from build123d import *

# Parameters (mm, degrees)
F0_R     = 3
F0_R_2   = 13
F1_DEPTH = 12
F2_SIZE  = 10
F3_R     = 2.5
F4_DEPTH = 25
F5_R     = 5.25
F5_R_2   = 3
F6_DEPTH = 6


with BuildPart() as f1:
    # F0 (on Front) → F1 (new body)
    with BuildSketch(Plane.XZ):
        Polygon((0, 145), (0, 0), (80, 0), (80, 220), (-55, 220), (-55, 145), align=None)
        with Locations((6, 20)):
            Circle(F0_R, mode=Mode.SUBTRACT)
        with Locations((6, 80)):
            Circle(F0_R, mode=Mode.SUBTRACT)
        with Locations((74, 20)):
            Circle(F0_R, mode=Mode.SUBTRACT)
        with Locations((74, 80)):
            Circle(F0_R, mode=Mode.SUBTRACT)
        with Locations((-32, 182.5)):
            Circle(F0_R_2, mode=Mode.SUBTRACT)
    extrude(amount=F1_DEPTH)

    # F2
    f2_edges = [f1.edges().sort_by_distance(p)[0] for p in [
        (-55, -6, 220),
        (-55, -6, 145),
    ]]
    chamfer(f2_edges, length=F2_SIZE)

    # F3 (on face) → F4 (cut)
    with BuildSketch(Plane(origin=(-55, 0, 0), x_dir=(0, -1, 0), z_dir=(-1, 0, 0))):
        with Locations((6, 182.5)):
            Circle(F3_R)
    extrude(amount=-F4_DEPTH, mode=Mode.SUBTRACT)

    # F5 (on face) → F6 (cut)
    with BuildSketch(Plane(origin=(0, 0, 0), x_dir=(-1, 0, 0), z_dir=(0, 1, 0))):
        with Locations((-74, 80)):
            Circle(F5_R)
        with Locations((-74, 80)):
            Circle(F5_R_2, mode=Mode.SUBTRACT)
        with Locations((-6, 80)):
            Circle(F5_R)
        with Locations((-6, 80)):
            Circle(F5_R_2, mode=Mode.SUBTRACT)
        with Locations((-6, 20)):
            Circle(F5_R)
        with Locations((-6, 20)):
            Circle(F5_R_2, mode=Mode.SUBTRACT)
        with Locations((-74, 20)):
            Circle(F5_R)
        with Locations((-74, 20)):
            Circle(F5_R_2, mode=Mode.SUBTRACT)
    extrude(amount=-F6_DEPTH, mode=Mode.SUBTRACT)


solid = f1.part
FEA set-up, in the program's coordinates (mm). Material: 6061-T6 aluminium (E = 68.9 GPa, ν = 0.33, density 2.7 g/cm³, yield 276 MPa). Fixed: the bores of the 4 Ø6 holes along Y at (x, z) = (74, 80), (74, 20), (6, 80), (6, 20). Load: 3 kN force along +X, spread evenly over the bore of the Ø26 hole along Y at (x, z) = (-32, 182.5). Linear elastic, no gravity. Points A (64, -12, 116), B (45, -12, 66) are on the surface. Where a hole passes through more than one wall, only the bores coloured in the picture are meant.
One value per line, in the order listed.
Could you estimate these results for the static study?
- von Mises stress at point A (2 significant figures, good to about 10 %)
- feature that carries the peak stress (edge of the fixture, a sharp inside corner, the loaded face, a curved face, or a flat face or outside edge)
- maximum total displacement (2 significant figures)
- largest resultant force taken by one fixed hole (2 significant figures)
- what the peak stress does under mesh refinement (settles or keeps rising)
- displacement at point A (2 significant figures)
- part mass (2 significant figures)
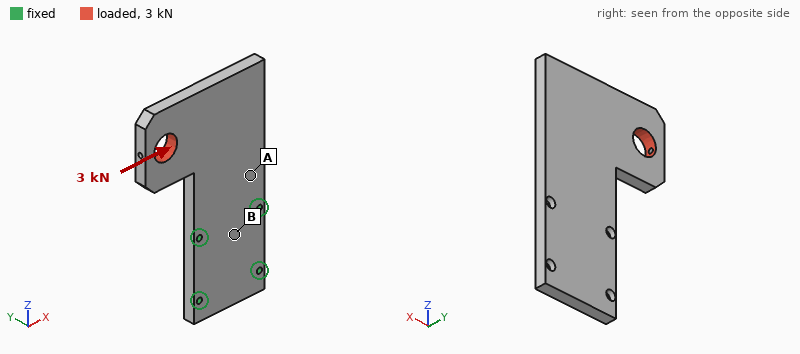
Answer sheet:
13 MPa
edge of the fixture
97 µm
4.2 kN
keeps rising
18 µm
680 g
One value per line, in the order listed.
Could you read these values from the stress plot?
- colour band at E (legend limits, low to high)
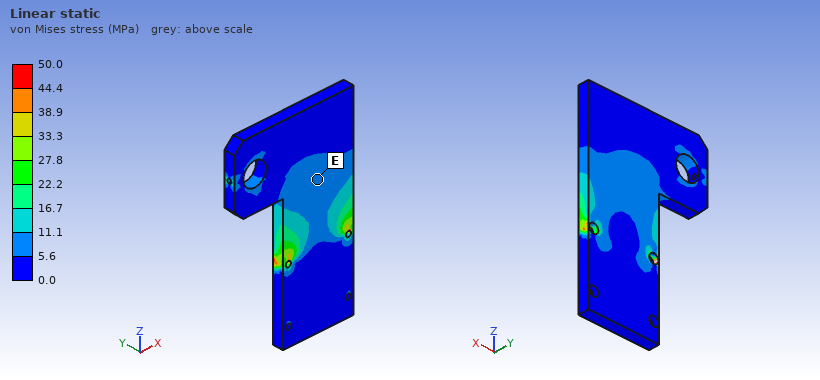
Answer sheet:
5.6 to 11.1 MPa
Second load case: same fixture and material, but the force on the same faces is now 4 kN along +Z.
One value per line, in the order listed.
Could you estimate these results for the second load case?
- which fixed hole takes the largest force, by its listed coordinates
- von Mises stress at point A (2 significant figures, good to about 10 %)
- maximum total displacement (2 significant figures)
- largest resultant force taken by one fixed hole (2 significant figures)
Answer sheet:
(6, 80)
11 MPa
0.14 mm
5.0 kN
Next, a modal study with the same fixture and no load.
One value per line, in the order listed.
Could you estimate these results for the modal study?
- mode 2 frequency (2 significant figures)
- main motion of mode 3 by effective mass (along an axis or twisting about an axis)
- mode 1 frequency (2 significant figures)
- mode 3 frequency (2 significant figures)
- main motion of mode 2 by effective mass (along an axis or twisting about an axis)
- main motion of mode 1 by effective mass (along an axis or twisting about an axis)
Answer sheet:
870 Hz
along X
330 Hz
1800 Hz
twisting about Z
along Y
